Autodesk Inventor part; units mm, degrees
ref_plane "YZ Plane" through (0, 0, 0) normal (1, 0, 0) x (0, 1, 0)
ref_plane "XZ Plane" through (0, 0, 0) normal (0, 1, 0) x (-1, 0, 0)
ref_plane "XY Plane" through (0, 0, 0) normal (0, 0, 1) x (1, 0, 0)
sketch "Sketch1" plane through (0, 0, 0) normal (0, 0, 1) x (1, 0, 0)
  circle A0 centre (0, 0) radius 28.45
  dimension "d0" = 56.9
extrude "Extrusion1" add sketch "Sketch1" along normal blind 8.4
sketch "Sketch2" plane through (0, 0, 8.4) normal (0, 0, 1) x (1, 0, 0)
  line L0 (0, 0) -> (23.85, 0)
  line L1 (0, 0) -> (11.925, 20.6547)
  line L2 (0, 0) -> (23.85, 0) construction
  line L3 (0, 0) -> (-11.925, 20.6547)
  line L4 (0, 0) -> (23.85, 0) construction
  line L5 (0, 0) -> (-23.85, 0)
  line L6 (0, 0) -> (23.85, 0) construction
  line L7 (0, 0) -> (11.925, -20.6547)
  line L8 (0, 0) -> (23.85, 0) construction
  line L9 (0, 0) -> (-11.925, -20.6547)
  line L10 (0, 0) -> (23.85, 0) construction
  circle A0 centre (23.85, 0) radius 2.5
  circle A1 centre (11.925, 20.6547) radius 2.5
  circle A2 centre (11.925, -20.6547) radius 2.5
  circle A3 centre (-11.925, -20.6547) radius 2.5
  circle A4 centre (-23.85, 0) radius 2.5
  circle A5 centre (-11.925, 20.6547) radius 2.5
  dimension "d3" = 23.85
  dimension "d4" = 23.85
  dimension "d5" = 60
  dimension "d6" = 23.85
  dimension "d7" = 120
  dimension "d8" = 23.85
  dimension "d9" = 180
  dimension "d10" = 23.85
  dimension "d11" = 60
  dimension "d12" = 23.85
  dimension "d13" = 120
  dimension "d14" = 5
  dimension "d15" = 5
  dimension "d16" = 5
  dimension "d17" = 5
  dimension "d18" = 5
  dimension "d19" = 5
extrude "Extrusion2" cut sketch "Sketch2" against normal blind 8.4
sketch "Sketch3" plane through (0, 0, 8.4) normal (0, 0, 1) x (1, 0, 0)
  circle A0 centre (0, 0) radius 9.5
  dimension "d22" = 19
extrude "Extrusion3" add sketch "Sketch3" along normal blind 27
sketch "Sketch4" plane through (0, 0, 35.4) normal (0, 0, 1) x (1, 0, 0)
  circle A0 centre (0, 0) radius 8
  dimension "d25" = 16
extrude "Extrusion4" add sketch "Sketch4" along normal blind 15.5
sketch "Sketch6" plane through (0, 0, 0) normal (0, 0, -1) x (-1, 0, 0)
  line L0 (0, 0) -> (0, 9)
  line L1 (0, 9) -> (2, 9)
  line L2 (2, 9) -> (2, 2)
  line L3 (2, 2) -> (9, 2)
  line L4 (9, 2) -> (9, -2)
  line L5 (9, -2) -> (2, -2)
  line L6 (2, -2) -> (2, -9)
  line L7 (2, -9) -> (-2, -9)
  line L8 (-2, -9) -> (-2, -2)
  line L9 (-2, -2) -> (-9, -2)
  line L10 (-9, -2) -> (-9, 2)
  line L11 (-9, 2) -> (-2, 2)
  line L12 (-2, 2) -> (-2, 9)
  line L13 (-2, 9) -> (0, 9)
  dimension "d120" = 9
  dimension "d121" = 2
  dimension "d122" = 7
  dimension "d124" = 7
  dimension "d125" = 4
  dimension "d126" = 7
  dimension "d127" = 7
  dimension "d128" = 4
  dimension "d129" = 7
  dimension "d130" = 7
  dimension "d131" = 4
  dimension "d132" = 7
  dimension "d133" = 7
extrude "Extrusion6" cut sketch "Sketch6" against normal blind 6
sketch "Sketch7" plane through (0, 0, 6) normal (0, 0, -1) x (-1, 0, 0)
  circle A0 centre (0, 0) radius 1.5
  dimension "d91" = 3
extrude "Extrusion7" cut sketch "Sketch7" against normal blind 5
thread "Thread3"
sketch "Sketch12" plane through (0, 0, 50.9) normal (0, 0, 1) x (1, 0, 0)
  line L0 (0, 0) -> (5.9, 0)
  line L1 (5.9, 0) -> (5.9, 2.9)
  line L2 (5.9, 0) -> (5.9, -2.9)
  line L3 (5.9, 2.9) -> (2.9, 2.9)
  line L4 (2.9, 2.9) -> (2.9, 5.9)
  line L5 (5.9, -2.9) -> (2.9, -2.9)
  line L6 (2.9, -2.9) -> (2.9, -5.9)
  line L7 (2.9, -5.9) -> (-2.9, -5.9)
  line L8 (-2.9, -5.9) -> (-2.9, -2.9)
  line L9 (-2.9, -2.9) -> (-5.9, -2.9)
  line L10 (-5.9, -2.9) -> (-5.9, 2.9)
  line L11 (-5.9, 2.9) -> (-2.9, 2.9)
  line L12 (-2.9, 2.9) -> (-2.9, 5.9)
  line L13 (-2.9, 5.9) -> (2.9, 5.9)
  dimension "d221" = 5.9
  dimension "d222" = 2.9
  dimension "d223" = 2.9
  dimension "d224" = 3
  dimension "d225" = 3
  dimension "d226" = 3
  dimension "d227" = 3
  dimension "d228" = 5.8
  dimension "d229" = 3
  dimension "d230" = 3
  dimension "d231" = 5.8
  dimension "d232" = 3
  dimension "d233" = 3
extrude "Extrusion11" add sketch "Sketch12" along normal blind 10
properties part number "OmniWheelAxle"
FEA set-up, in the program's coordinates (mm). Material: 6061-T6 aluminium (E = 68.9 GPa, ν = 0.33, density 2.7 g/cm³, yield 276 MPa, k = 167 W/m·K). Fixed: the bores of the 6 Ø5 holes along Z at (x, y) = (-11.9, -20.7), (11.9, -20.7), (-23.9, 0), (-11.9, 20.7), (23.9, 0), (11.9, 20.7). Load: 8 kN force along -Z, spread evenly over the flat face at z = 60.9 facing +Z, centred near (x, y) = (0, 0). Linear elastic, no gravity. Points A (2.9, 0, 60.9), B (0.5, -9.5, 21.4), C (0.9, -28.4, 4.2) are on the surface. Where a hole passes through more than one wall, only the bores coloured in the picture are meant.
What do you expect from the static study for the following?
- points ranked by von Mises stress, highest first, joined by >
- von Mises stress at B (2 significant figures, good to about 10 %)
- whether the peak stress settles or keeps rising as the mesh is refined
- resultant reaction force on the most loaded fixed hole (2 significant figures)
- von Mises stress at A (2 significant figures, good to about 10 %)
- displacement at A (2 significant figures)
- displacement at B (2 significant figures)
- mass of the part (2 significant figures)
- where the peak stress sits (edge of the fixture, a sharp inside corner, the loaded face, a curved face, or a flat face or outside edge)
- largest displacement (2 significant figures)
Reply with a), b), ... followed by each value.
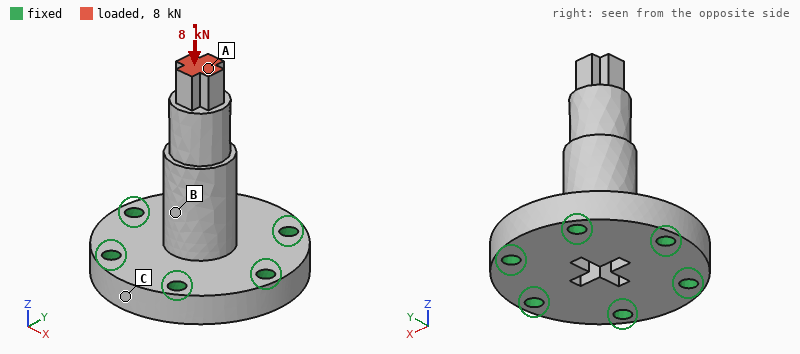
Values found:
a) A > B > C
b) 27 MPa
c) keeps rising
d) 1.6 kN
e) 78 MPa
f) 54 µm
g) 27 µm
h) 85 g
i) edge of the fixture
j) 54 µm
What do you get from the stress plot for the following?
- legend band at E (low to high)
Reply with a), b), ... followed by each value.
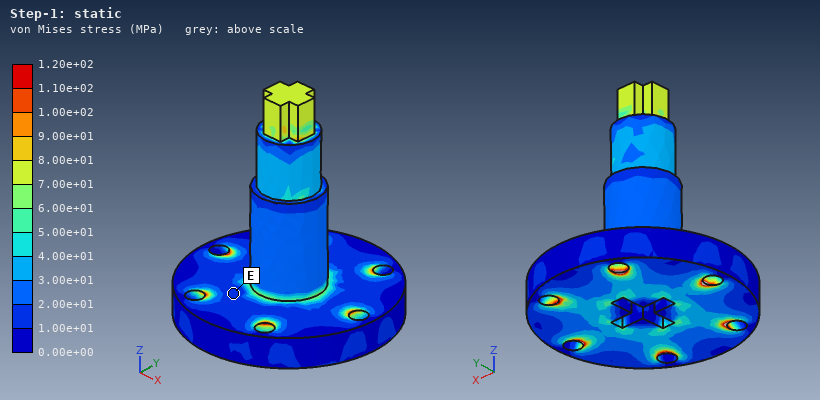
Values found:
a) 1.00e+01 to 2.00e+01 MPa
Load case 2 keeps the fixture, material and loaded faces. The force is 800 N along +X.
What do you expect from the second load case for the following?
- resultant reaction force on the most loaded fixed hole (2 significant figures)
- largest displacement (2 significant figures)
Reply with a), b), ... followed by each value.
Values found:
a) 870 N
b) 0.18 mm
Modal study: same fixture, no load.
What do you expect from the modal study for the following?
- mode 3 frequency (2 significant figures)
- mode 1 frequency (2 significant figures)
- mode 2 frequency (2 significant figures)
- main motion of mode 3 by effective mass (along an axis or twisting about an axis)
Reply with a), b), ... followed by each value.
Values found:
a) 14 kHz
b) 4400 Hz
c) 4400 Hz
d) along Z
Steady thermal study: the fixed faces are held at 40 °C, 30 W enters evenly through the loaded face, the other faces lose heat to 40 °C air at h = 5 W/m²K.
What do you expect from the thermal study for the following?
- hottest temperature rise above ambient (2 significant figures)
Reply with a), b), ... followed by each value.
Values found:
a) 55 K
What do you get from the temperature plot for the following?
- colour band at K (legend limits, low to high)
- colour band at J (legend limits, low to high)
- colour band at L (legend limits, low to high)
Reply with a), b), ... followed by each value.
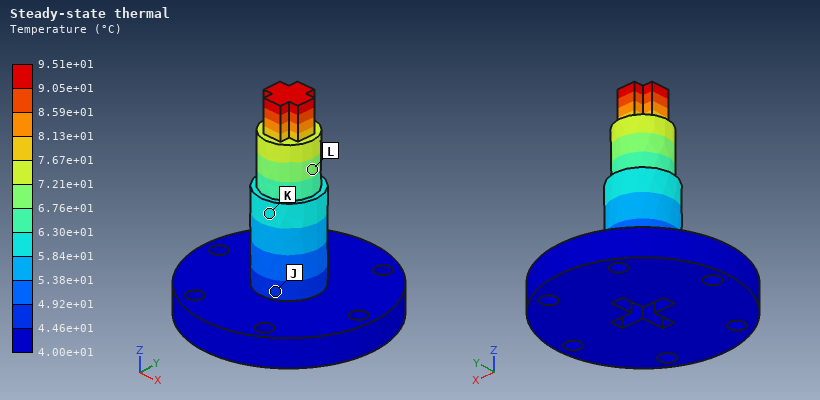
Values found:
a) 5.84e+01 to 6.30e+01 °C
b) 4.46e+01 to 4.92e+01 °C
c) 6.76e+01 to 7.21e+01 °C
